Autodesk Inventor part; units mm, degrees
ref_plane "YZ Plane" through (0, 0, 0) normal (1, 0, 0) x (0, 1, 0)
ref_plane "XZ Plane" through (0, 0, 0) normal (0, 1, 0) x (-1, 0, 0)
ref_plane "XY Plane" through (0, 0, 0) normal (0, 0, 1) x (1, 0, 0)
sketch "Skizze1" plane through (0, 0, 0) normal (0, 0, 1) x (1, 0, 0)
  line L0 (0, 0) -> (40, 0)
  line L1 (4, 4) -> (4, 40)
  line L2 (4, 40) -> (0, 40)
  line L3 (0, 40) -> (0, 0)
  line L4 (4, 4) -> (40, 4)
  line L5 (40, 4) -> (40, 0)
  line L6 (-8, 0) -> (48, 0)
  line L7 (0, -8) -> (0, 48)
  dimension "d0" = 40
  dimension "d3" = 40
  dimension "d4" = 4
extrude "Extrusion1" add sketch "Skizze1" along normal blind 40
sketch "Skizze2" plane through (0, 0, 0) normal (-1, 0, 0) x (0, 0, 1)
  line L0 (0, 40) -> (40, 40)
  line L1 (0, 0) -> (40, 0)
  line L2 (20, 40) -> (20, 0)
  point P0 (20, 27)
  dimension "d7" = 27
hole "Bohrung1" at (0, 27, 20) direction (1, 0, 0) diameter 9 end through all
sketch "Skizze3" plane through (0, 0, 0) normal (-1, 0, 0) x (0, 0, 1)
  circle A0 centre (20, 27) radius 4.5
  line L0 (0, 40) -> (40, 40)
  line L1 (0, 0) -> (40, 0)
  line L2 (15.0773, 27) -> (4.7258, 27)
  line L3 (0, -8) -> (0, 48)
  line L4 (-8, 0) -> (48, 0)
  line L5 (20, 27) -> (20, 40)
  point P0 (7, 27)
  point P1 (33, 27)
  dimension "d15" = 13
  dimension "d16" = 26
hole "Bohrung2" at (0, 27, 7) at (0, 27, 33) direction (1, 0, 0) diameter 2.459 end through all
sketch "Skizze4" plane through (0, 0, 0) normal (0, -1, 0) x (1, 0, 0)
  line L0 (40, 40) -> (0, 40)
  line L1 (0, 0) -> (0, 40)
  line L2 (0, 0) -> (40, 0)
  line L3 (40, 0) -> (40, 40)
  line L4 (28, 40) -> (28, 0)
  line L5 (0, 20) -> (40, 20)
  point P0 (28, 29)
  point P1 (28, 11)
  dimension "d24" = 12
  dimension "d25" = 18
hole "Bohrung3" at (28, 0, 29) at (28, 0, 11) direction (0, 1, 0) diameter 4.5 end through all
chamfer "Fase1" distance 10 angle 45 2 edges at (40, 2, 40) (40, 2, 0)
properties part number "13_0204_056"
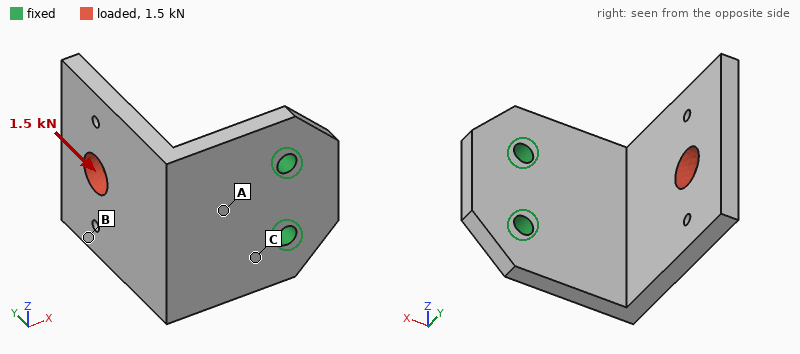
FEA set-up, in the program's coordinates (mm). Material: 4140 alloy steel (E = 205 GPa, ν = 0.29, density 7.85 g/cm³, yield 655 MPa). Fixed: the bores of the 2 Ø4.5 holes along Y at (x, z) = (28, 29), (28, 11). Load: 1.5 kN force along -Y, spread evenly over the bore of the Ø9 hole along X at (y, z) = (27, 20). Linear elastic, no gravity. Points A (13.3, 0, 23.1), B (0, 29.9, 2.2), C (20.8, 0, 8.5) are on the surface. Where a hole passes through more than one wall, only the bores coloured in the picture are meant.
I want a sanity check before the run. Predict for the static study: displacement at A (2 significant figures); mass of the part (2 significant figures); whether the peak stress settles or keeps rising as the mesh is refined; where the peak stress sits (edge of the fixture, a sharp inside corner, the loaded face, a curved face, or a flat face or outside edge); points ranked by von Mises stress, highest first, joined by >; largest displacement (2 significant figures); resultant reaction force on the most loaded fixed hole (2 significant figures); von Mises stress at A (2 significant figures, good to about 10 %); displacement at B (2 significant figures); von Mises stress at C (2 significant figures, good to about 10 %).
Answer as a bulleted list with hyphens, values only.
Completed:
- 0.077 mm
- 89 g
- keeps rising
- edge of the fixture
- C > A > B
- 0.47 mm
- 750 N
- 140 MPa
- 0.37 mm
- 250 MPa
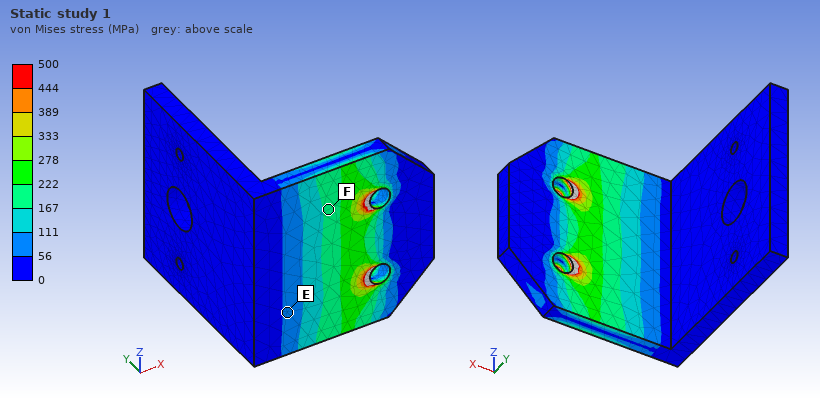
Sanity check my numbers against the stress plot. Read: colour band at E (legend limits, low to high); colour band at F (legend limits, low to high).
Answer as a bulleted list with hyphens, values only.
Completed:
- 56 to 111 MPa
- 167 to 222 MPa
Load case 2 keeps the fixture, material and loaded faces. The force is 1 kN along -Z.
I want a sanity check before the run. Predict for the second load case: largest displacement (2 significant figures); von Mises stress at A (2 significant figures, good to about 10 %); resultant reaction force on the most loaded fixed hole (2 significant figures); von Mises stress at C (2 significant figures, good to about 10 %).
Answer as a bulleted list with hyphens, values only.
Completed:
- 0.25 mm
- 130 MPa
- 1.6 kN
- 130 MPa
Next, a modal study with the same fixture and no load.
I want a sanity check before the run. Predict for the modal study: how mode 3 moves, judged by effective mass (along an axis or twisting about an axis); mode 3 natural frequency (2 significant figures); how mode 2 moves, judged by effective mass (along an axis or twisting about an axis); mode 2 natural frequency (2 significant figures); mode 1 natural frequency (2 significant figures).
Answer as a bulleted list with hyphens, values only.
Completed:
- along Y
- 3200 Hz
- along Z
- 2000 Hz
- 1100 Hz
